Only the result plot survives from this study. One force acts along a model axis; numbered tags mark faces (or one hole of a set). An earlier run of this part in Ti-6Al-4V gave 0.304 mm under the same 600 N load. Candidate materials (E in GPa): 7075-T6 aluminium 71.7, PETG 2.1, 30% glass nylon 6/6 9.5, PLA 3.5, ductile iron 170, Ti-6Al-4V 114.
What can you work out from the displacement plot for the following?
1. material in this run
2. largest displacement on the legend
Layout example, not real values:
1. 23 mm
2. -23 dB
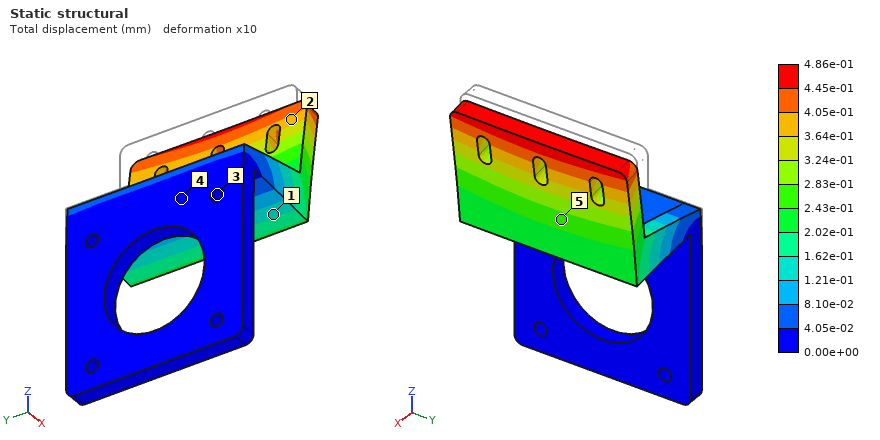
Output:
1. 7075-T6 aluminium
2. 4.86e-01 mm
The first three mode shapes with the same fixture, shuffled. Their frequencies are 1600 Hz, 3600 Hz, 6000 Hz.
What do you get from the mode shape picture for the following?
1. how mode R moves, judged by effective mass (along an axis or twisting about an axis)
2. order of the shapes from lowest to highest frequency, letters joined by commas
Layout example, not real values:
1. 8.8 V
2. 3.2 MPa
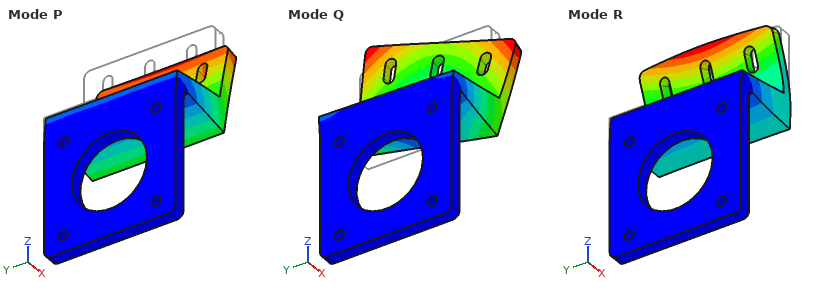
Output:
1. along Z
2. P, Q, R
